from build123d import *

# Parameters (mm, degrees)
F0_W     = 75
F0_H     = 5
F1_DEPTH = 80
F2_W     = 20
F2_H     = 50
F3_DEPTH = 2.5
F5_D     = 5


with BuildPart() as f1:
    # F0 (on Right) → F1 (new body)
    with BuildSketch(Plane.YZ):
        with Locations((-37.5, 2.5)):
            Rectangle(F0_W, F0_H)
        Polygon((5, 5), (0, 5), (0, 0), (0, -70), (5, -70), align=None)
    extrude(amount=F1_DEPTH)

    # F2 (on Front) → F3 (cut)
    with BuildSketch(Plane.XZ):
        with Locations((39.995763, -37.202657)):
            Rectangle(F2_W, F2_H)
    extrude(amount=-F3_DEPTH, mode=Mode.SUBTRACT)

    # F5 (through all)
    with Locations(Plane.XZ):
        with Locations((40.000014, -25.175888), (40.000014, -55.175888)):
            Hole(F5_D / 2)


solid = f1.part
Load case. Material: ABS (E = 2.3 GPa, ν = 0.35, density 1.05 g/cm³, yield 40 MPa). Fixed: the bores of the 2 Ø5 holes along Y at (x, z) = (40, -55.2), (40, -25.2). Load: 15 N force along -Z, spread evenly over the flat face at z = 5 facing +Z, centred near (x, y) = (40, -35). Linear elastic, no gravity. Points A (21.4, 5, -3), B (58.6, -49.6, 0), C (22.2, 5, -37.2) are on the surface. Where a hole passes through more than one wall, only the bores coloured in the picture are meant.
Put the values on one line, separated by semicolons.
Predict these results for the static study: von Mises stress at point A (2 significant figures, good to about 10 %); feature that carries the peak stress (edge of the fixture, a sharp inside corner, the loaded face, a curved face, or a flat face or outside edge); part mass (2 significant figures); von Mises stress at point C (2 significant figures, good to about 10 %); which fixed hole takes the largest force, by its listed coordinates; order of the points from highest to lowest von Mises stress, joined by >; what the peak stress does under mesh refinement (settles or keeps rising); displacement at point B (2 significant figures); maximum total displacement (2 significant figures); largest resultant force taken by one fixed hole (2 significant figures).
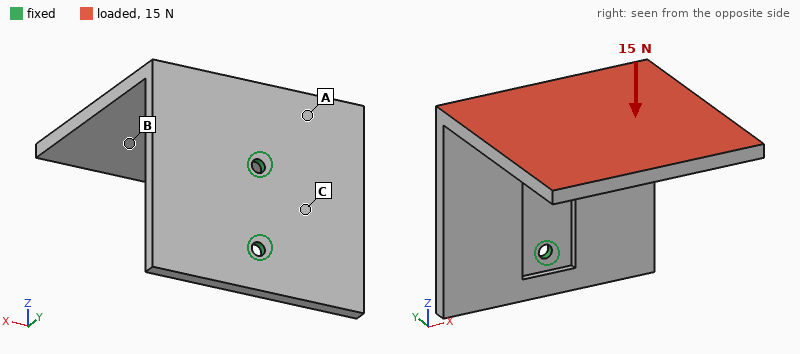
1.5 MPa; edge of the fixture; 60 g; 0.85 MPa; (40, -55.2); A > C > B; keeps rising; 0.92 mm; 1.4 mm; 26 N
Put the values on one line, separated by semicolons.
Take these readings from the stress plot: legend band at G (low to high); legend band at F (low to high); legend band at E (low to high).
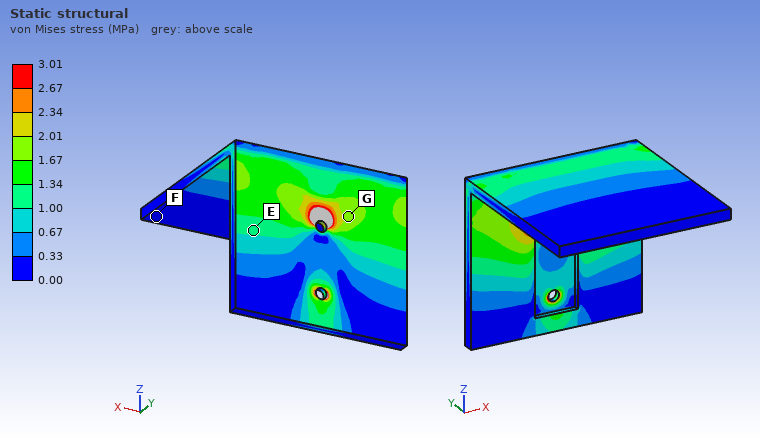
1.67 to 2.01 MPa; 0.00 to 0.33 MPa; 1.00 to 1.34 MPa
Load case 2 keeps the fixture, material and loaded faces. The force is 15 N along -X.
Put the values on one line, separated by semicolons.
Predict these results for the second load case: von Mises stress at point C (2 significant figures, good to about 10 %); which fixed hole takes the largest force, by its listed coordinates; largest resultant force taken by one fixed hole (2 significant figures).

1.2 MPa; (40, -25.2); 28 N
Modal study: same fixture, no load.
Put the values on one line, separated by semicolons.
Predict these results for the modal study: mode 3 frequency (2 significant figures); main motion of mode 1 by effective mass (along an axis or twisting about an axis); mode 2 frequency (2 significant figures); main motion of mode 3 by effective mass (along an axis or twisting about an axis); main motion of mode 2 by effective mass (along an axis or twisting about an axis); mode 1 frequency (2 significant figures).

350 Hz; along X; 100 Hz; along Y; along Z; 98 Hz
